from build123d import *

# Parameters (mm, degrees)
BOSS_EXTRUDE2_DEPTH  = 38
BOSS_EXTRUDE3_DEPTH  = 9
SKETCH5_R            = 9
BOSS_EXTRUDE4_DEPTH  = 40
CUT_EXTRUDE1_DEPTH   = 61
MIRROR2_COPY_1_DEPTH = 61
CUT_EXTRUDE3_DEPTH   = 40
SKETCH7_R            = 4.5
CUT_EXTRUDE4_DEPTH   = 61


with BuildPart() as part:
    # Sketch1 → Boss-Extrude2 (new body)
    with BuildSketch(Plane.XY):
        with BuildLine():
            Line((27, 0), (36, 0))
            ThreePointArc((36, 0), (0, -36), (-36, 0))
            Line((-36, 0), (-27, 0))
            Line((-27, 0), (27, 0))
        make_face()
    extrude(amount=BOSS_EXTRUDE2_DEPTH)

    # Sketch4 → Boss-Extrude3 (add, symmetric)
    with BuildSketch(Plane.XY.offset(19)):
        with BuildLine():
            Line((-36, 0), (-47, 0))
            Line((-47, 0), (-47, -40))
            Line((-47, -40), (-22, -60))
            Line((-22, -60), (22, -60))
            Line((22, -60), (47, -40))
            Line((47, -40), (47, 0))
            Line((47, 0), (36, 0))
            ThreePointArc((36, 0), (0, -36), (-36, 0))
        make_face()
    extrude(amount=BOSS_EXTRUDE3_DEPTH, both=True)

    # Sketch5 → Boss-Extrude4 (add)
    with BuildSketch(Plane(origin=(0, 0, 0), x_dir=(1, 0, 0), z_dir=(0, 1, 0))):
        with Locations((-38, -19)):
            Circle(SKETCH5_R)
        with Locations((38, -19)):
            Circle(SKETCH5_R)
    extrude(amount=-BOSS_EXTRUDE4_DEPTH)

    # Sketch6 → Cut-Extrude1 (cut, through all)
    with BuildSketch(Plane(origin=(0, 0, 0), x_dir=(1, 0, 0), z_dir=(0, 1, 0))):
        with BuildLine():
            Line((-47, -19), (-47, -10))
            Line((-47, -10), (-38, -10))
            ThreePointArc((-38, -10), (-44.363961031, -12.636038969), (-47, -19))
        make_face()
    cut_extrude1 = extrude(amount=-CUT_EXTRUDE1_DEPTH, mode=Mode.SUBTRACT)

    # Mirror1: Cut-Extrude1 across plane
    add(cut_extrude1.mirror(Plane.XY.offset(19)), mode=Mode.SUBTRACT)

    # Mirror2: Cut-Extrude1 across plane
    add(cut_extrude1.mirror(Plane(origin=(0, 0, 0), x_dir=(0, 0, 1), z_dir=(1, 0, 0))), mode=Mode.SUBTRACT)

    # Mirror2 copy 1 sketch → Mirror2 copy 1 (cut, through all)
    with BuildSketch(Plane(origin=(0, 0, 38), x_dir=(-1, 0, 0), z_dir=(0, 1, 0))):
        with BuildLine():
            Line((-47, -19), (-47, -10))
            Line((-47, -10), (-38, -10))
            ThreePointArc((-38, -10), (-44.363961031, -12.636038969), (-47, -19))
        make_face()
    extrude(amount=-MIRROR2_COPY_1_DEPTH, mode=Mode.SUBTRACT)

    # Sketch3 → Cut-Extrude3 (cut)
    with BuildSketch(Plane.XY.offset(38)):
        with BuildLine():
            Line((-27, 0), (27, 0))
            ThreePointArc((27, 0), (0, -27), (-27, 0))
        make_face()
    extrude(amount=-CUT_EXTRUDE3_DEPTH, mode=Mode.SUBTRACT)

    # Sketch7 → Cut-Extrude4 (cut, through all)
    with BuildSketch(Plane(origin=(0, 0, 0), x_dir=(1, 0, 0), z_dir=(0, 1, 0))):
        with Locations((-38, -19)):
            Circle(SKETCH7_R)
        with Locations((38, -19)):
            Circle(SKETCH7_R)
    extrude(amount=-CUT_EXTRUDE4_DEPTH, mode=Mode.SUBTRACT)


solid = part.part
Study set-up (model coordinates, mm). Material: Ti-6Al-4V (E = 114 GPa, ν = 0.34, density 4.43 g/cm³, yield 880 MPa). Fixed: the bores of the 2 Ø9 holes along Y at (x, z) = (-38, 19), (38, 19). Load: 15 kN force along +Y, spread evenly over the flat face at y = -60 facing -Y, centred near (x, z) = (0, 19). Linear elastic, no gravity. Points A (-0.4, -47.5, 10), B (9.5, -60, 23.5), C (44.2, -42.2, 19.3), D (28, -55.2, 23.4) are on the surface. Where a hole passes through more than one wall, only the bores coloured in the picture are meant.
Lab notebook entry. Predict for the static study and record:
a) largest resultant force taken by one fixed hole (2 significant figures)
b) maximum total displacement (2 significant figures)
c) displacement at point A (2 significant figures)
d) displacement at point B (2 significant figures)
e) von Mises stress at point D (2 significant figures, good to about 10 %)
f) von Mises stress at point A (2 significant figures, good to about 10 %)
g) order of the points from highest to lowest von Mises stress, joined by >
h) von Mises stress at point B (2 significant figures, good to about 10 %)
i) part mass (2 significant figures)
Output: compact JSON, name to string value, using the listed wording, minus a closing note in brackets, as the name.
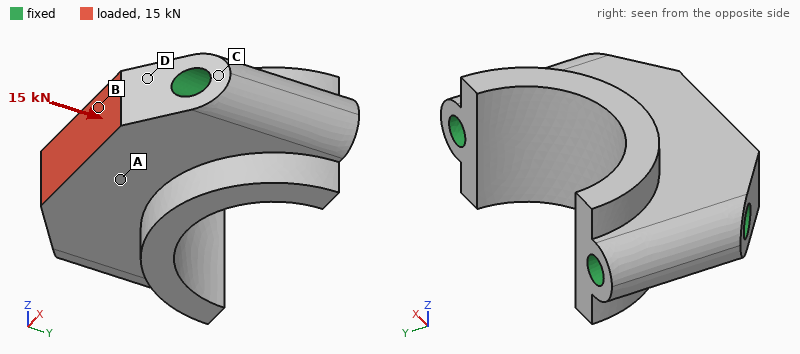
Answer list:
{"largest resultant force taken by one fixed hole": "8.7 kN", "maximum total displacement": "9.5 µm", "displacement at point A": "8.1 µm", "displacement at point B": "8.7 µm", "von Mises stress at point D": "9.4 MPa", "von Mises stress at point A": "14 MPa", "order of the points from highest to lowest von Mises stress, joined by >": "B > A > D > C", "von Mises stress at point B": "21 MPa", "part mass": "360 g"}
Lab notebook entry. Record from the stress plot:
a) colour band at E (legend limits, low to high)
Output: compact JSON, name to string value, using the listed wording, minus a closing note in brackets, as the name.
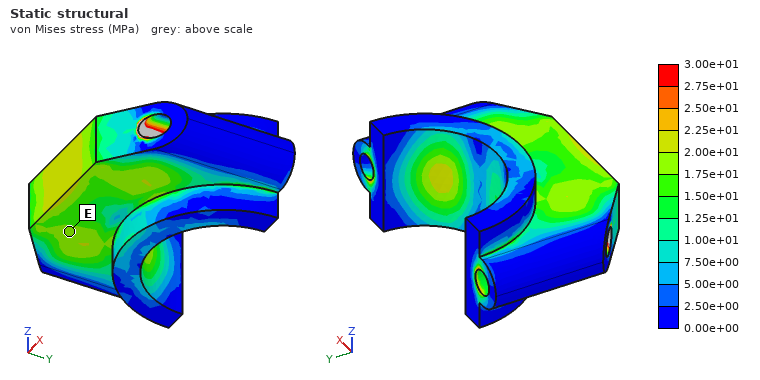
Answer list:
{"colour band at E": "1.75e+01 to 2.00e+01 MPa"}
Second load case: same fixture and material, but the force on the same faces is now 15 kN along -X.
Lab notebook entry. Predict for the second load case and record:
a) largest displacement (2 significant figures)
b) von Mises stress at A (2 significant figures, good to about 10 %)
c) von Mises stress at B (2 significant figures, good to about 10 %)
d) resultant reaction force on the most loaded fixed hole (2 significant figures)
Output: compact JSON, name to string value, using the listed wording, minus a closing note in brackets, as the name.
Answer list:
{"largest displacement": "8.5 µm", "von Mises stress at A": "17 MPa", "von Mises stress at B": "33 MPa", "resultant reaction force on the most loaded fixed hole": "8.9 kN"}
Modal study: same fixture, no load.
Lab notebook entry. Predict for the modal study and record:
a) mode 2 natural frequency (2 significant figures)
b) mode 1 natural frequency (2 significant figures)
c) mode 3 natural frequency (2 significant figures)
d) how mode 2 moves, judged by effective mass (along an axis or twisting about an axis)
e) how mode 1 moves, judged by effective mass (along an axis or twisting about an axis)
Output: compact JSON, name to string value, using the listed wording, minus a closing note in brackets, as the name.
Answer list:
{"mode 2 natural frequency": "19 kHz", "mode 1 natural frequency": "11 kHz", "mode 3 natural frequency": "20 kHz", "how mode 2 moves, judged by effective mass": "along Y", "how mode 1 moves, judged by effective mass": "along Z"}
